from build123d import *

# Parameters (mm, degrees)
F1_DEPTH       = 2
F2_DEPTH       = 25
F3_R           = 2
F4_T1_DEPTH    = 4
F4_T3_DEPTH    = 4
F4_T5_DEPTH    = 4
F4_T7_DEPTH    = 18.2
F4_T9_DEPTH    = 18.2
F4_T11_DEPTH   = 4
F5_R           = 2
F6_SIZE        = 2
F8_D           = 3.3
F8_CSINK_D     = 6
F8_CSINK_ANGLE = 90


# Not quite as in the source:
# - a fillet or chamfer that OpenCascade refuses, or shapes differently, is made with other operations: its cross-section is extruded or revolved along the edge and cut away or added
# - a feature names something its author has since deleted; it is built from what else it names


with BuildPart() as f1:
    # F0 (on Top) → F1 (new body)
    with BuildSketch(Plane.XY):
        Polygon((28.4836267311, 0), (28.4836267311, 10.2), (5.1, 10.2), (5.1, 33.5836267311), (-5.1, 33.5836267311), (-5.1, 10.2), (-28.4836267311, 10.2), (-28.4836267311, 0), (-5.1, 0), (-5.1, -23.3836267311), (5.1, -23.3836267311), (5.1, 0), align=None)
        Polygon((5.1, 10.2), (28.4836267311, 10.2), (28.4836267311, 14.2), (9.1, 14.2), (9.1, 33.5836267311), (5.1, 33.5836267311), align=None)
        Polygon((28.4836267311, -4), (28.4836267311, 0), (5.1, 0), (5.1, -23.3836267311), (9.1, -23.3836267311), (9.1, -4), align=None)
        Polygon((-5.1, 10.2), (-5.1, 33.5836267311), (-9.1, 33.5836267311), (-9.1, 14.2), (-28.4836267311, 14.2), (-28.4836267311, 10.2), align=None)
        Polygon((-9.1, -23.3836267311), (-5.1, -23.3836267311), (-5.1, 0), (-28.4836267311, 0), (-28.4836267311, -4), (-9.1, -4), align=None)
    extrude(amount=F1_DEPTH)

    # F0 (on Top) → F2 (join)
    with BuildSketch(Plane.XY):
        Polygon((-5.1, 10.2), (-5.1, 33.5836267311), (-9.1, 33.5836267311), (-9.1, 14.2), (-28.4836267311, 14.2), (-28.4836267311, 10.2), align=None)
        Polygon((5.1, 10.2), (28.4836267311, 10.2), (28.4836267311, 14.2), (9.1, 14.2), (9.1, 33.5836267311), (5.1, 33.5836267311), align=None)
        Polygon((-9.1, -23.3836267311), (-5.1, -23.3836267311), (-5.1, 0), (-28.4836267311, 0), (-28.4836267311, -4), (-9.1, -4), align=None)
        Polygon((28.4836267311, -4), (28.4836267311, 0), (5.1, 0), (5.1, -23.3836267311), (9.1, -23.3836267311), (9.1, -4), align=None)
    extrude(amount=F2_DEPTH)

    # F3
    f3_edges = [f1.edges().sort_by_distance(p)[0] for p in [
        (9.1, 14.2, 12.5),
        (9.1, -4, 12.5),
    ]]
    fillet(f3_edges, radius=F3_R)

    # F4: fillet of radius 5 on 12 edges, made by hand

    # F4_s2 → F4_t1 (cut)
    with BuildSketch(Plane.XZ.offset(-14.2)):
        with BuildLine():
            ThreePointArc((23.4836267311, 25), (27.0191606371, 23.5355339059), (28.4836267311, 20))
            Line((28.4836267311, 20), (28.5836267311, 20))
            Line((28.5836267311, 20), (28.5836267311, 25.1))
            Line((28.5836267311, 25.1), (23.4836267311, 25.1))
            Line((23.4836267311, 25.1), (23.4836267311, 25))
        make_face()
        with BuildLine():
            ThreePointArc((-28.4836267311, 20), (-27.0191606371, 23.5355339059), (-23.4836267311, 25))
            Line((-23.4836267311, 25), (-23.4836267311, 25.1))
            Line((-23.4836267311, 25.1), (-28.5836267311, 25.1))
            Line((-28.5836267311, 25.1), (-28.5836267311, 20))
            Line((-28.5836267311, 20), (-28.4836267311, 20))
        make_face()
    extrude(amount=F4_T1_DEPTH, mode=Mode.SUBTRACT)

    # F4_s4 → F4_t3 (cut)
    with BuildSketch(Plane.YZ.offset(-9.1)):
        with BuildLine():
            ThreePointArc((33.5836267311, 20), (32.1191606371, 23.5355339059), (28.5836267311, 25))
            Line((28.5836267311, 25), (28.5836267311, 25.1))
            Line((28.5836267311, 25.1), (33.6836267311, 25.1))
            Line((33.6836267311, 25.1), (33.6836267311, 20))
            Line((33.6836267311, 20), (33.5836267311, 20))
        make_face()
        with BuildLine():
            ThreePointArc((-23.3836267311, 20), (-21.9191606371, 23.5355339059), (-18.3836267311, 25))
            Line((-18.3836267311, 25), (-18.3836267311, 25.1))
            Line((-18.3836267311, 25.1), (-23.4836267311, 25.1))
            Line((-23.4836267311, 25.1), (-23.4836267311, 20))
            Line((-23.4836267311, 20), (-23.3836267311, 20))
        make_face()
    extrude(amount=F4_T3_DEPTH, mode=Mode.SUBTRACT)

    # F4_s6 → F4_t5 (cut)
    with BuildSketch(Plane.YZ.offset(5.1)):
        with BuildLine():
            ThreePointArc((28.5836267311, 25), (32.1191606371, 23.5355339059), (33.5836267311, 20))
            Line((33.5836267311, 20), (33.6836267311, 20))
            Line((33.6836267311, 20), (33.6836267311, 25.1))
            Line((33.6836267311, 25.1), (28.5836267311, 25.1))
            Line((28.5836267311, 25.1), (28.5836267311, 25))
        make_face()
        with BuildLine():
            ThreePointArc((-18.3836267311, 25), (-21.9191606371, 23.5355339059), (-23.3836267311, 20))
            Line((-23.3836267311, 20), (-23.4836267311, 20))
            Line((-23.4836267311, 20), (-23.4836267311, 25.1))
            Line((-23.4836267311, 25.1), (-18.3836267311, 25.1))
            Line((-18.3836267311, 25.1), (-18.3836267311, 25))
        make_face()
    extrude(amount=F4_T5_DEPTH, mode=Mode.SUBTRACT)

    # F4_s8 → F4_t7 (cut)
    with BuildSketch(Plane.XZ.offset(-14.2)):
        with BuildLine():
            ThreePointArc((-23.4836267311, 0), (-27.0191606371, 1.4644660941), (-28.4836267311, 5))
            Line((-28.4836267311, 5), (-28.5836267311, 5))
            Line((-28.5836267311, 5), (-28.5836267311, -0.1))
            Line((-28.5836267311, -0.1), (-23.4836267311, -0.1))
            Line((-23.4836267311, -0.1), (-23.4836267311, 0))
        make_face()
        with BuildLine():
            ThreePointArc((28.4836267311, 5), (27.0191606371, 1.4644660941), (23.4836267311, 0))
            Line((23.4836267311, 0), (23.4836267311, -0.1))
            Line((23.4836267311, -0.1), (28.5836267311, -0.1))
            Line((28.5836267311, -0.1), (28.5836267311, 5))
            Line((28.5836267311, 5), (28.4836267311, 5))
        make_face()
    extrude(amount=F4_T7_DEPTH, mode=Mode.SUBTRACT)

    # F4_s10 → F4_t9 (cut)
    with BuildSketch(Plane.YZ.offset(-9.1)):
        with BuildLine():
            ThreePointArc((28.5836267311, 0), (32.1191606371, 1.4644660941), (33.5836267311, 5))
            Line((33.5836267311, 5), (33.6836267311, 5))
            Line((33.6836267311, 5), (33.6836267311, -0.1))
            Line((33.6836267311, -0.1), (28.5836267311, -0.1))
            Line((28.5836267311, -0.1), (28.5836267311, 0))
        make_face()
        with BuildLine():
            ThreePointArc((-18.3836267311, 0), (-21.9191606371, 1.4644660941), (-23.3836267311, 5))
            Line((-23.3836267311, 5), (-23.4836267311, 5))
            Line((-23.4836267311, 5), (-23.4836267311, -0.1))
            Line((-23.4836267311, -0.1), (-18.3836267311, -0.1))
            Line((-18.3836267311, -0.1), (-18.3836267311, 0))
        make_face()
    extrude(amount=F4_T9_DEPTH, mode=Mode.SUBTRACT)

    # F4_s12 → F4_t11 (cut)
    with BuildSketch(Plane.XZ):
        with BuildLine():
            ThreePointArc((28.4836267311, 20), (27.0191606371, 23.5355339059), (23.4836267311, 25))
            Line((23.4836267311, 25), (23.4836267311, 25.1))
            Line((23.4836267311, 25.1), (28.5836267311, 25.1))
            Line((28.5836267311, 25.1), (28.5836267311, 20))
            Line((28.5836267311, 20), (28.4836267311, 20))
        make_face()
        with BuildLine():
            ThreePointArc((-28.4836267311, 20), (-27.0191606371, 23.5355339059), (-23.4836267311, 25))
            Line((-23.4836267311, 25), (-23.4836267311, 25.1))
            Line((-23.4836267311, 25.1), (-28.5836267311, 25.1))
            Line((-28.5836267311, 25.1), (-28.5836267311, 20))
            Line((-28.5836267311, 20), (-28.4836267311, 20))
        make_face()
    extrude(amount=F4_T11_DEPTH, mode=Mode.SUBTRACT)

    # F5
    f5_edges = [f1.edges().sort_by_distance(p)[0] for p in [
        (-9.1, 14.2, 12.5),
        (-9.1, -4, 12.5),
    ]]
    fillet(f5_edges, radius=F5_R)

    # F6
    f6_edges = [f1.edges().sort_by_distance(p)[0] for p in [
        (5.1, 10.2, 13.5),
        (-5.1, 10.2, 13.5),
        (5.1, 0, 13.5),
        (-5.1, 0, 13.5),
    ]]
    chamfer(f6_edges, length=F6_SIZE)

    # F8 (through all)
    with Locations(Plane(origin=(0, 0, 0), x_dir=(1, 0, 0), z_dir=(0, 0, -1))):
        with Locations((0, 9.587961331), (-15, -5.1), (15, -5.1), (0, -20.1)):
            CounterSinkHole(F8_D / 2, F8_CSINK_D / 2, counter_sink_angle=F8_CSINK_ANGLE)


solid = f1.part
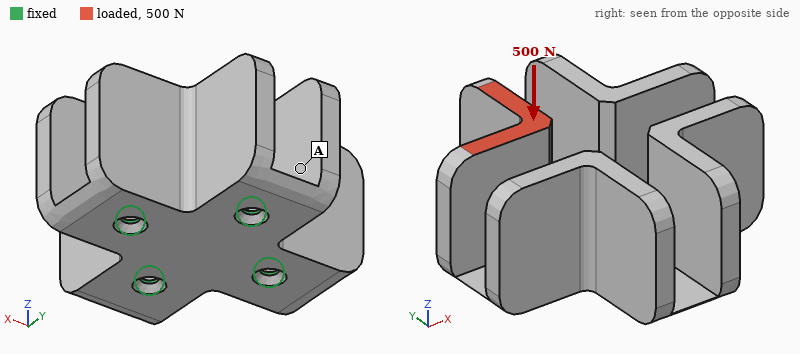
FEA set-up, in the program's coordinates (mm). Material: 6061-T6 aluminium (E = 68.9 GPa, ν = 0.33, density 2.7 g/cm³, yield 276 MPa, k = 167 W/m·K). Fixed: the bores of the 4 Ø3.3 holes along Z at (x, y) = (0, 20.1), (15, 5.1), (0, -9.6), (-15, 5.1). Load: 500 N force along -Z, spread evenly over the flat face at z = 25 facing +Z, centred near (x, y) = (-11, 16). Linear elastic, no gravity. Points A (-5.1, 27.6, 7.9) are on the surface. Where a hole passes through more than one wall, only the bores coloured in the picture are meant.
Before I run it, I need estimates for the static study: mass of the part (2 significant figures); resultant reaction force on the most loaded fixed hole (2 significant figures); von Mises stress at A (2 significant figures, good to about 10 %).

50 g
300 N
11 MPa
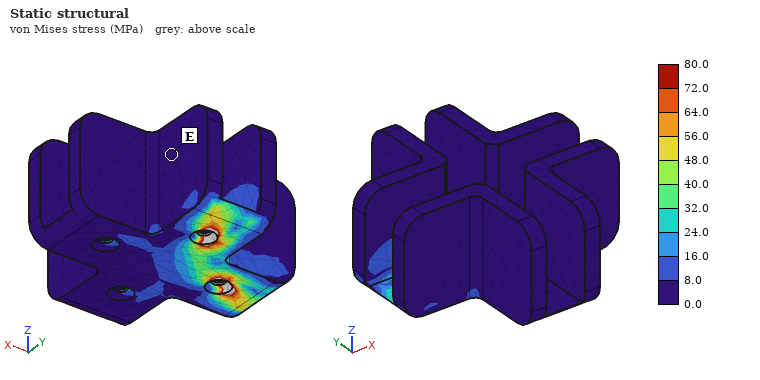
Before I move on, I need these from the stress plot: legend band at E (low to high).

0.0 to 8.0 MPa
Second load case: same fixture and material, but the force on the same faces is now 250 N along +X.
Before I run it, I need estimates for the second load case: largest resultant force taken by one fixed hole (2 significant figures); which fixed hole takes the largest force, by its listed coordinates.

440 N
(-15, 5.1)
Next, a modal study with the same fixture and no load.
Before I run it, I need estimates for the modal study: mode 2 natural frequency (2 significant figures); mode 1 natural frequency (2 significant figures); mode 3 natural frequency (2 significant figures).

2300 Hz
1800 Hz
2300 Hz
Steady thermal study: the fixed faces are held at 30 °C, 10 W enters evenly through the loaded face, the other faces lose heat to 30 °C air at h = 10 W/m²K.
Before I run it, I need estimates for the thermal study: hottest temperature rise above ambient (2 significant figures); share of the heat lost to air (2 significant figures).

16 K
3.8 %
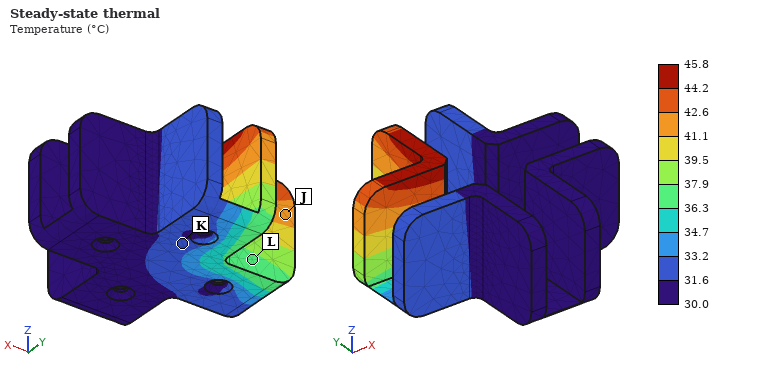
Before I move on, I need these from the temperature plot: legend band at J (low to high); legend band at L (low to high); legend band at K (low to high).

41.1 to 42.6 °C
36.3 to 37.9 °C
31.6 to 33.2 °C
